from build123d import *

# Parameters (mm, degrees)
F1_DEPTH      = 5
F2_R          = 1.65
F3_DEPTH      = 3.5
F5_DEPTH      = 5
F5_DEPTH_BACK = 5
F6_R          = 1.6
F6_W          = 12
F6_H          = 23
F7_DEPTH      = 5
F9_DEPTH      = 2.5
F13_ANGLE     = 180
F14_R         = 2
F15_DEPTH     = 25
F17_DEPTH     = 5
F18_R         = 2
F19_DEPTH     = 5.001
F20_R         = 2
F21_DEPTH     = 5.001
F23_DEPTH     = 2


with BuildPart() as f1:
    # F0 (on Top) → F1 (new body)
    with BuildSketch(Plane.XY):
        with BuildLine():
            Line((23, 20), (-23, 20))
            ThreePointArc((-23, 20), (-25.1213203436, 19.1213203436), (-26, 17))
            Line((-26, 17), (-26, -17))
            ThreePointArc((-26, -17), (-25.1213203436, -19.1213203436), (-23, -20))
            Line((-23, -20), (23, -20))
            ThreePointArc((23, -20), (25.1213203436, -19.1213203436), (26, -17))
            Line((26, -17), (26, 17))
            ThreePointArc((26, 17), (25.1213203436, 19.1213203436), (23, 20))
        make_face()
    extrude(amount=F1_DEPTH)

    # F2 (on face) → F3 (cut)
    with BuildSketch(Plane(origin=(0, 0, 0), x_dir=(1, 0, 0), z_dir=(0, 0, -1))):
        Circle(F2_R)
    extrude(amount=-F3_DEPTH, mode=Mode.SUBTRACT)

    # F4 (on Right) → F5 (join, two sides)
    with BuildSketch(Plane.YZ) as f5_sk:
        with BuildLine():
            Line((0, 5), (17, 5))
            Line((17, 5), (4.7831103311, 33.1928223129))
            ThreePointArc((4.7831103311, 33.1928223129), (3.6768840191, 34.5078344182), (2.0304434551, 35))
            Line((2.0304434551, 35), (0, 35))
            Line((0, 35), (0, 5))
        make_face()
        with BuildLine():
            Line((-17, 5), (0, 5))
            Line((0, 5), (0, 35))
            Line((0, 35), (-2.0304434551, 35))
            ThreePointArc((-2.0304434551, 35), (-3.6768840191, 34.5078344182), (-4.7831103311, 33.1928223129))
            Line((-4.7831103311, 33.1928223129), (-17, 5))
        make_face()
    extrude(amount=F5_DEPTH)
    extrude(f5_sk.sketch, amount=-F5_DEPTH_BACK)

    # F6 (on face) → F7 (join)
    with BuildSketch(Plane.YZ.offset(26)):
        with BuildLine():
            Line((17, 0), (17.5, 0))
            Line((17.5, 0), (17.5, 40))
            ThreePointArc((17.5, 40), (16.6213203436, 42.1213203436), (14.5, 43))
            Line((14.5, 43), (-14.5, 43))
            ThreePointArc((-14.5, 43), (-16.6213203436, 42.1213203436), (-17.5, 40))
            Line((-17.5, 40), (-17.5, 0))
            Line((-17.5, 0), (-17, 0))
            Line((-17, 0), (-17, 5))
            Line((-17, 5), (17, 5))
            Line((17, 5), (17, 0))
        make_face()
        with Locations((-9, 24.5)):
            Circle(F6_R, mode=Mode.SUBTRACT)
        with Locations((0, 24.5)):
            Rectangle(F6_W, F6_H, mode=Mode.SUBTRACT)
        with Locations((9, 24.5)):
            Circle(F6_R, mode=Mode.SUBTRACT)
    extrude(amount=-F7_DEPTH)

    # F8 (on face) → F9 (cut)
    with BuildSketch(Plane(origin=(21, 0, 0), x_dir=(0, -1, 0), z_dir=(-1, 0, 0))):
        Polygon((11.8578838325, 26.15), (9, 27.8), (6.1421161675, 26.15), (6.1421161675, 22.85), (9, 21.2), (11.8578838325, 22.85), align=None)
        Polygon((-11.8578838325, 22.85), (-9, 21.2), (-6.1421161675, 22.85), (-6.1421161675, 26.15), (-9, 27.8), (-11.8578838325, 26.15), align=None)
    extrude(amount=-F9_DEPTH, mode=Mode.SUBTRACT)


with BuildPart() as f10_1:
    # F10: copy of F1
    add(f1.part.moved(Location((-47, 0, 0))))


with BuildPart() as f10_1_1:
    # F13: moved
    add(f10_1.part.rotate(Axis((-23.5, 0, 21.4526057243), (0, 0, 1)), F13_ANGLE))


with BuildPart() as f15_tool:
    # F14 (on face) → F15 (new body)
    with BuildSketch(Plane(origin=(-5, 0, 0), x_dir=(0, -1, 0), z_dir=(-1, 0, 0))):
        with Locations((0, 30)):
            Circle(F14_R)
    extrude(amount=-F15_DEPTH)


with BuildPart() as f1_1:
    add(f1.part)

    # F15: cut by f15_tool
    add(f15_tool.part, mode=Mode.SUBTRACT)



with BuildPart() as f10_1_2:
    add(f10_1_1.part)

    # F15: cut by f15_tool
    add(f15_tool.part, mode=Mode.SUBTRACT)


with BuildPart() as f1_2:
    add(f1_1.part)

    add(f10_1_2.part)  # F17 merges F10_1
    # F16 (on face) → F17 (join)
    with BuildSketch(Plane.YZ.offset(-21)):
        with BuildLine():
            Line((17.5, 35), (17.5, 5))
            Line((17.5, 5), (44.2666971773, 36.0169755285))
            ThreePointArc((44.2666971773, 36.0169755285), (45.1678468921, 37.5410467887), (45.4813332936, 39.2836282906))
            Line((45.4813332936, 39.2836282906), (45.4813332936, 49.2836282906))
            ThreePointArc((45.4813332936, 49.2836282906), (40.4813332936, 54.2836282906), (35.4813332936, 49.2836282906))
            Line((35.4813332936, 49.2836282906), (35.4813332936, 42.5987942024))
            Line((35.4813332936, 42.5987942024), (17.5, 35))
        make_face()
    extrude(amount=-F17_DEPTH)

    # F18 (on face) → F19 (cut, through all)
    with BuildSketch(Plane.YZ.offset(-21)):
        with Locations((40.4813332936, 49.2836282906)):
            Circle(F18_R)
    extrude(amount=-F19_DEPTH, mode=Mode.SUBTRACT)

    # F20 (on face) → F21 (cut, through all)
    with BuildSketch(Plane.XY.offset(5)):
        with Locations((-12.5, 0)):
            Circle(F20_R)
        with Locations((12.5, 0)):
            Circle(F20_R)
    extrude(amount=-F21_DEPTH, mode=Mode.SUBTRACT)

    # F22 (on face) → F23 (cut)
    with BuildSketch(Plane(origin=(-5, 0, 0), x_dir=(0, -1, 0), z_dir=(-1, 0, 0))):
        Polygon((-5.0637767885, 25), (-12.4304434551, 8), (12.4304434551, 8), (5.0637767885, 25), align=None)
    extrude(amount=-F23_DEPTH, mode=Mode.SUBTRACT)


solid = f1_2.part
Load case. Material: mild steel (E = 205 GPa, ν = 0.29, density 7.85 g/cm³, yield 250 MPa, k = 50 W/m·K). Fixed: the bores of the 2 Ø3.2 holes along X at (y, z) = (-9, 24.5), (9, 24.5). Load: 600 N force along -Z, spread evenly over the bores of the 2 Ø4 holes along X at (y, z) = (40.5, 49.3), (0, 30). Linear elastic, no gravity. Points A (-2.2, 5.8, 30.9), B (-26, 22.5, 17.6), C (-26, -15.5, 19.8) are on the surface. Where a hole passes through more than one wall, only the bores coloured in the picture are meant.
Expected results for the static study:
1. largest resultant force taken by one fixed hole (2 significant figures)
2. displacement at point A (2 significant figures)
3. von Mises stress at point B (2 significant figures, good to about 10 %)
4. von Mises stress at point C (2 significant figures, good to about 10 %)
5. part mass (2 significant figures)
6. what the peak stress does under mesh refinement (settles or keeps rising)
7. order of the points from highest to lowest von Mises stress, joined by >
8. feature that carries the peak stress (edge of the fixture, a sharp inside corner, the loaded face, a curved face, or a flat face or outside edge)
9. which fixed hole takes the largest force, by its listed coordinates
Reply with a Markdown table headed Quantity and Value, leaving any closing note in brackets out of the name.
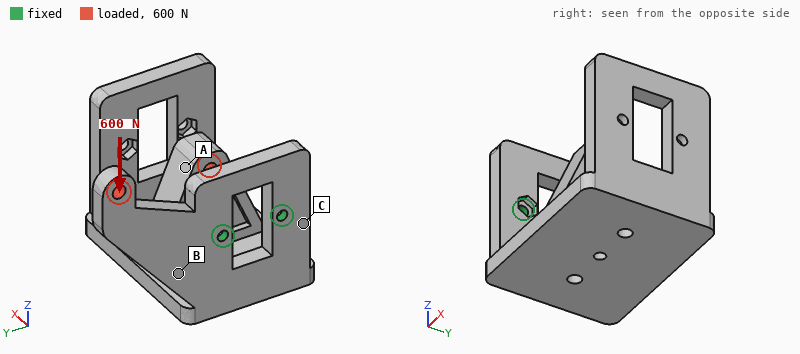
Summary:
| Quantity | Value |
|---|---|
| largest resultant force taken by one fixed hole | 620 N |
| displacement at point A | 0.16 mm |
| von Mises stress at point B | 48 MPa |
| von Mises stress at point C | 90 MPa |
| part mass | 230 g |
| what the peak stress does under mesh refinement | keeps rising |
| order of the points from highest to lowest von Mises stress, joined by > | C > B > A |
| feature that carries the peak stress | edge of the fixture |
| which fixed hole takes the largest force, by its listed coordinates | (9, 24.5) |
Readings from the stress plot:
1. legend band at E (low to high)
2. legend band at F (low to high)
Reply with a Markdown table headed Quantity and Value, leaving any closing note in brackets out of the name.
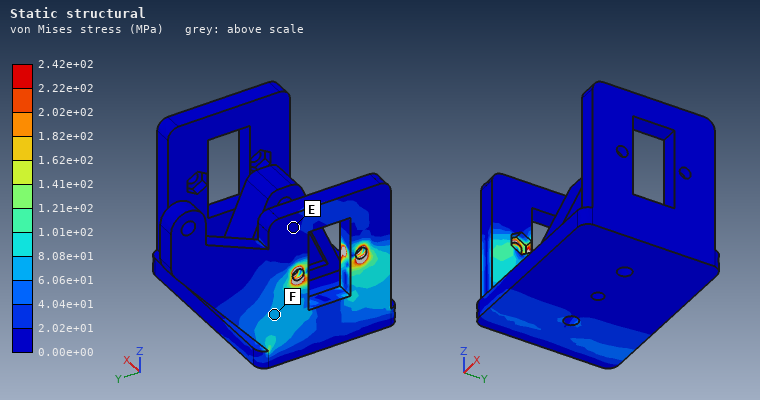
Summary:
| Quantity | Value |
|---|---|
| legend band at E | 0.00e+00 to 2.02e+01 MPa |
| legend band at F | 6.06e+01 to 8.08e+01 MPa |
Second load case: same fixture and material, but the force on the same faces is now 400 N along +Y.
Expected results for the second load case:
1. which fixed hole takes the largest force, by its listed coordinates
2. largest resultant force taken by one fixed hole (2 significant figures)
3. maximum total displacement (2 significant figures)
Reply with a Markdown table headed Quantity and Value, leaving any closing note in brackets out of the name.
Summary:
| Quantity | Value |
|---|---|
| which fixed hole takes the largest force, by its listed coordinates | (9, 24.5) |
| largest resultant force taken by one fixed hole | 400 N |
| maximum total displacement | 0.11 mm |
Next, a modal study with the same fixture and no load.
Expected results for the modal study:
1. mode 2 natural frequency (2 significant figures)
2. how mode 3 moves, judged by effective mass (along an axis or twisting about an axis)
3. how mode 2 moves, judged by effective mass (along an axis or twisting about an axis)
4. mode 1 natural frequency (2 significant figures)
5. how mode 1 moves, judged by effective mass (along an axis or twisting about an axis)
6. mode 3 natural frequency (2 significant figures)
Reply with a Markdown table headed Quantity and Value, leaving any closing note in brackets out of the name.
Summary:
| Quantity | Value |
|---|---|
| mode 2 natural frequency | 790 Hz |
| how mode 3 moves, judged by effective mass | along X |
| how mode 2 moves, judged by effective mass | along Y |
| mode 1 natural frequency | 430 Hz |
| how mode 1 moves, judged by effective mass | along Z |
| mode 3 natural frequency | 1300 Hz |
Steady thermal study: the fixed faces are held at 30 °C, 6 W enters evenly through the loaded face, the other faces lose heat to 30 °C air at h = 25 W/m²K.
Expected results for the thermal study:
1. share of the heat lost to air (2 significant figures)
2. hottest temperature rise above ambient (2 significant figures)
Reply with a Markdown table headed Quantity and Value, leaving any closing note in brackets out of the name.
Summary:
| Quantity | Value |
|---|---|
| share of the heat lost to air | 52 % |
| hottest temperature rise above ambient | 25 K |
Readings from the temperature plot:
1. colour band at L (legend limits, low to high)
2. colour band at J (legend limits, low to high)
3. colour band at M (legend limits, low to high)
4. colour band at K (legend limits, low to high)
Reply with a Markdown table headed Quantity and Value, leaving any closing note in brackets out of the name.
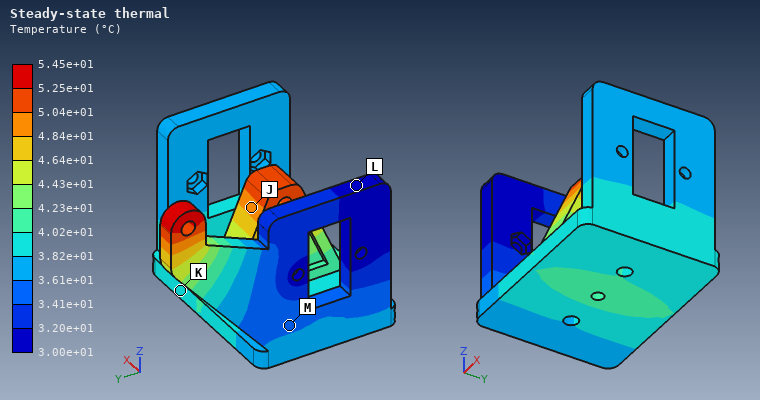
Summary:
| Quantity | Value |
|---|---|
| colour band at L | 3.00e+01 to 3.20e+01 °C |
| colour band at J | 4.84e+01 to 5.04e+01 °C |
| colour band at M | 3.41e+01 to 3.61e+01 °C |
| colour band at K | 3.82e+01 to 4.02e+01 °C |
